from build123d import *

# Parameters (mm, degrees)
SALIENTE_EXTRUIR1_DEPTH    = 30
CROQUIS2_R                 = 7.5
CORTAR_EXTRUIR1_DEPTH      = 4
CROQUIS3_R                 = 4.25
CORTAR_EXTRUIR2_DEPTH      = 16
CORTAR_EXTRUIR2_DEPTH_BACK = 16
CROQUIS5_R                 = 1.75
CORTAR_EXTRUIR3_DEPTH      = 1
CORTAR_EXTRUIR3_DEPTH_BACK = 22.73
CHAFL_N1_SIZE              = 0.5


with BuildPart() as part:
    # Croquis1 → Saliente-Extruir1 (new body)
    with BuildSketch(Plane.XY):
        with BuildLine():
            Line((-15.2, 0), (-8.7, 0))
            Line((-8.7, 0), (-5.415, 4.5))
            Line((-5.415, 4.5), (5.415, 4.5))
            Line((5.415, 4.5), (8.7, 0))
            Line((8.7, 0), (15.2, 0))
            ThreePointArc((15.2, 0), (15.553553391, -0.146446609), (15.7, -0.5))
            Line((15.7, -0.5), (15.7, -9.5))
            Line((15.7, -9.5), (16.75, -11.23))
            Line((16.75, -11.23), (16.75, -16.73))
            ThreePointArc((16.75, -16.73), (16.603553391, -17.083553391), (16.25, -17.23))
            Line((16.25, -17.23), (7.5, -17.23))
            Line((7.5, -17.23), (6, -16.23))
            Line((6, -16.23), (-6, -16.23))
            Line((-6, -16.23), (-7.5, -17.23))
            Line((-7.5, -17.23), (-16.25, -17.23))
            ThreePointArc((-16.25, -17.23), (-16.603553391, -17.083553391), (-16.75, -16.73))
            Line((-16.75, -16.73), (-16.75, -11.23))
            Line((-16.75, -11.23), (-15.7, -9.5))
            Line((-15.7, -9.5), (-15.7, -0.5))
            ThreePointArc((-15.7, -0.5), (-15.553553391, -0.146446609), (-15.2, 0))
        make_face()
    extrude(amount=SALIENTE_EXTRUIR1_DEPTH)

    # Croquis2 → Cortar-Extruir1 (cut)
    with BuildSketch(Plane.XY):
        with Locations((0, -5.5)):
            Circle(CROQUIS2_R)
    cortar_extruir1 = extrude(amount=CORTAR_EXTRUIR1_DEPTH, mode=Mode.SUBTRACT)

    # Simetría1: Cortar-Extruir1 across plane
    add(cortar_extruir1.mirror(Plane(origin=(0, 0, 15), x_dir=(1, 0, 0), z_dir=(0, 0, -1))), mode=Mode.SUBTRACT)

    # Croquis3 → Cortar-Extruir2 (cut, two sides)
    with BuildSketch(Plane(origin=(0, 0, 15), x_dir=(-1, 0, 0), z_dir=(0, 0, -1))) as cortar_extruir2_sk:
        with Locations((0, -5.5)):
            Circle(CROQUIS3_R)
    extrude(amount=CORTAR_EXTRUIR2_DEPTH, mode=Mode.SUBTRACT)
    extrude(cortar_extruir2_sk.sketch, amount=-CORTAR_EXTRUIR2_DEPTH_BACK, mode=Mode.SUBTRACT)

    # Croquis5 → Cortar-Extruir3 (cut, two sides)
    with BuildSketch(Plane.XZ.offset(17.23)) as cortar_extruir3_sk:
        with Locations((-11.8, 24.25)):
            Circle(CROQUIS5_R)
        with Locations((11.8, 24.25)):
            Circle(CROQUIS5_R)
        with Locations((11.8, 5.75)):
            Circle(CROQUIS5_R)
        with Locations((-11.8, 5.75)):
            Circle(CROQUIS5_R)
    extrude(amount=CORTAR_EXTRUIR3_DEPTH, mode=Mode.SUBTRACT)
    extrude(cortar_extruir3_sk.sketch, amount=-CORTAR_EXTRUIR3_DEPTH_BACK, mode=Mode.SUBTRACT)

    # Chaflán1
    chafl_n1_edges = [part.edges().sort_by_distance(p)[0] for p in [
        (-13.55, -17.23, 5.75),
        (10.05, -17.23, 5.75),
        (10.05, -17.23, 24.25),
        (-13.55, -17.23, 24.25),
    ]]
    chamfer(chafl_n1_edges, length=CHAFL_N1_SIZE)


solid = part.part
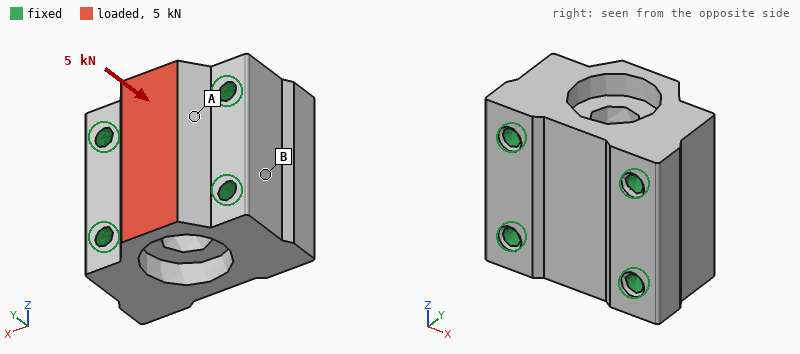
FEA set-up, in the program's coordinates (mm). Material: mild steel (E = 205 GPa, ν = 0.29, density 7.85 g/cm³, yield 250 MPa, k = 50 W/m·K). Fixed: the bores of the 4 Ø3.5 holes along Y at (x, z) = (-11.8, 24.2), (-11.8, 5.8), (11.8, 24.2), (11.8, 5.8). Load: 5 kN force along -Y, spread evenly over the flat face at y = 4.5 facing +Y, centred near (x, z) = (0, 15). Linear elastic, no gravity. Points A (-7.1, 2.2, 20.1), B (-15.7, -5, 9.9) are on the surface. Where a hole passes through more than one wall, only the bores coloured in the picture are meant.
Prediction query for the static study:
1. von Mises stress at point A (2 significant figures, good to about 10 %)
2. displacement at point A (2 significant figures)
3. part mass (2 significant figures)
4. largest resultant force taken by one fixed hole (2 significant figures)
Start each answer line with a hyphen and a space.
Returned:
- 15 MPa
- 0.71 µm
- 120 g
- 1.4 kN
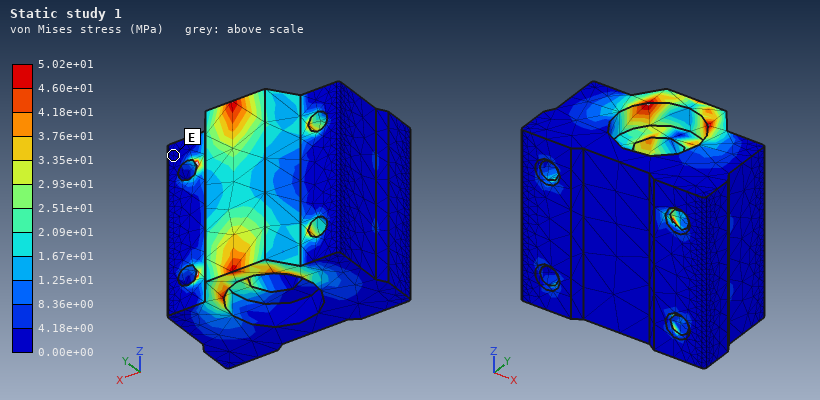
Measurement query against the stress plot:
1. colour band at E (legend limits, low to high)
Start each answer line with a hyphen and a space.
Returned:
- 0.00e+00 to 4.18e+00 MPa
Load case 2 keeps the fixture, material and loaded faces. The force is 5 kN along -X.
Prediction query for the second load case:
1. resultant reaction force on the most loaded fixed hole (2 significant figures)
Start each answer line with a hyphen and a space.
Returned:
- 1.6 kN
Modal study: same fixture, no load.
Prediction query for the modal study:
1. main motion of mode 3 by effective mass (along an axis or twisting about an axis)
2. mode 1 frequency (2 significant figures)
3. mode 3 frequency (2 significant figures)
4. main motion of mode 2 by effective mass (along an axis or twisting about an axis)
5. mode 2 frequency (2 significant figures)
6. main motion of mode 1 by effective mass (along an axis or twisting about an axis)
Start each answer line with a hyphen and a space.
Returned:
- along X
- 53 kHz
- 67 kHz
- along Y
- 57 kHz
- along Z
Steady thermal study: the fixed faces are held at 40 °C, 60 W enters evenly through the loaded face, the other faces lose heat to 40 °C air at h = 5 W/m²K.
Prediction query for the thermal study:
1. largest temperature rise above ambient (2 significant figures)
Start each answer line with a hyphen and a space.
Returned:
- 49 K
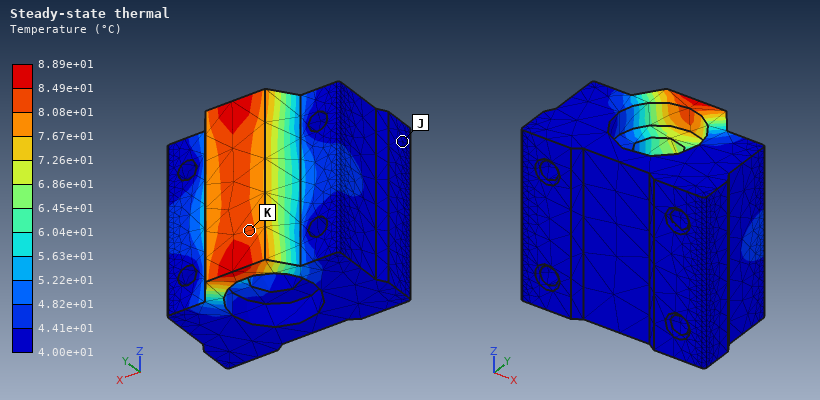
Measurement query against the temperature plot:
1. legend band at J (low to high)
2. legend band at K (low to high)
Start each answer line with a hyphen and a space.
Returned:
- 4.00e+01 to 4.41e+01 °C
- 8.08e+01 to 8.49e+01 °C
